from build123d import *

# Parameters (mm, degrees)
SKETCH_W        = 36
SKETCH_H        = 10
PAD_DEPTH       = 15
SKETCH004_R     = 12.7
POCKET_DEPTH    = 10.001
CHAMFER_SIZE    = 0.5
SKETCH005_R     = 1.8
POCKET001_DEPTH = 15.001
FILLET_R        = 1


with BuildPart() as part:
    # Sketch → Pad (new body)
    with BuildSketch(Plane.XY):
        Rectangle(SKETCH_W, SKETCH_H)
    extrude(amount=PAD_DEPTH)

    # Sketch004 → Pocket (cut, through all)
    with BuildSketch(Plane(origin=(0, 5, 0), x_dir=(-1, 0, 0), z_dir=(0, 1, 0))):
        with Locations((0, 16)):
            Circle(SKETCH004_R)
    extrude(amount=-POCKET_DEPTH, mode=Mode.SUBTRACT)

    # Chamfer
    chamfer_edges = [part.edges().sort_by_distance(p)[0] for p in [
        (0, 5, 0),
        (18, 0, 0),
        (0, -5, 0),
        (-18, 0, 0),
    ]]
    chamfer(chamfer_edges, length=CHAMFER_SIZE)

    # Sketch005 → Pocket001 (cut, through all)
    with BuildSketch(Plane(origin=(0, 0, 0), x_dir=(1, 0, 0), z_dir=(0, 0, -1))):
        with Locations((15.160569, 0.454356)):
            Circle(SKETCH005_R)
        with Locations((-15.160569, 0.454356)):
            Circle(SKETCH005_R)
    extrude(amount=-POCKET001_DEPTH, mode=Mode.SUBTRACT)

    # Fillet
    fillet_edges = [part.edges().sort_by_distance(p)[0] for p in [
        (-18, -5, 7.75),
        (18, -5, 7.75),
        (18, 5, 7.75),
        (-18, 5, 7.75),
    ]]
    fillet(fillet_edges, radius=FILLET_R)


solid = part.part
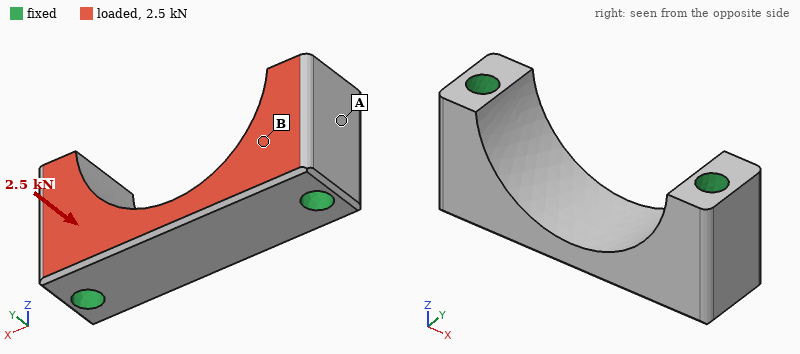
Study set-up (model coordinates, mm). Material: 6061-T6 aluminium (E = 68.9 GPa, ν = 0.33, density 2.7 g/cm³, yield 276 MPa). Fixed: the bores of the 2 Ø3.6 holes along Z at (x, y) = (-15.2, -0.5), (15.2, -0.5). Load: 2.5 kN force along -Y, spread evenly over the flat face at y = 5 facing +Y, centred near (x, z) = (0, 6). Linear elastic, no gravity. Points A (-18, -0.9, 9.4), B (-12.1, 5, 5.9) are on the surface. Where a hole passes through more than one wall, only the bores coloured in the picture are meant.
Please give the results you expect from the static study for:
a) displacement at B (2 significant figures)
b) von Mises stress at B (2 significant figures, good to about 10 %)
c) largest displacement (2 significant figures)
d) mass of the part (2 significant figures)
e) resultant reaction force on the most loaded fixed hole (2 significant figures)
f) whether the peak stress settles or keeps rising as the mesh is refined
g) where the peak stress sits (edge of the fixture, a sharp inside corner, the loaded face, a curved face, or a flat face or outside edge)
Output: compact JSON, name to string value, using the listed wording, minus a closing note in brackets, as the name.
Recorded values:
{"displacement at B": "2.7 µm", "von Mises stress at B": "16 MPa", "largest displacement": "7.5 µm", "mass of the part": "7.5 g", "resultant reaction force on the most loaded fixed hole": "1.3 kN", "whether the peak stress settles or keeps rising as the mesh is refined": "keeps rising", "where the peak stress sits": "edge of the fixture"}
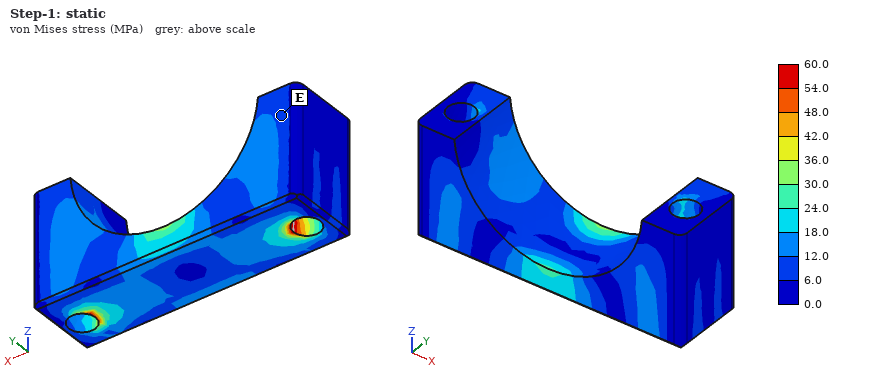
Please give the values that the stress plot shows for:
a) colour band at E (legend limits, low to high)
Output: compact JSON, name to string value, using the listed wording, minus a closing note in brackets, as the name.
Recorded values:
{"colour band at E": "6.0 to 12.0 MPa"}
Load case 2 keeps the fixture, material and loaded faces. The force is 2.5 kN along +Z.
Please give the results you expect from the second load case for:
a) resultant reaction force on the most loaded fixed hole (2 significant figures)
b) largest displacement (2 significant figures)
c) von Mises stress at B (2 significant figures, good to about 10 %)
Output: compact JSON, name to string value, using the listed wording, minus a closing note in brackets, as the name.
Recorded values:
{"resultant reaction force on the most loaded fixed hole": "1.3 kN", "largest displacement": "14 µm", "von Mises stress at B": "27 MPa"}
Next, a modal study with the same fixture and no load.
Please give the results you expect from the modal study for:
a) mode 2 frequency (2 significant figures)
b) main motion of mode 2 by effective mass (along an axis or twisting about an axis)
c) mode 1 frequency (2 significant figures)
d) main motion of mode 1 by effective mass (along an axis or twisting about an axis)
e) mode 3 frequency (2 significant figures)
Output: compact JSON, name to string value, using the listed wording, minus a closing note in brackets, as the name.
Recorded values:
{"mode 2 frequency": "46 kHz", "main motion of mode 2 by effective mass": "along Z", "mode 1 frequency": "39 kHz", "main motion of mode 1 by effective mass": "along Y", "mode 3 frequency": "69 kHz"}
